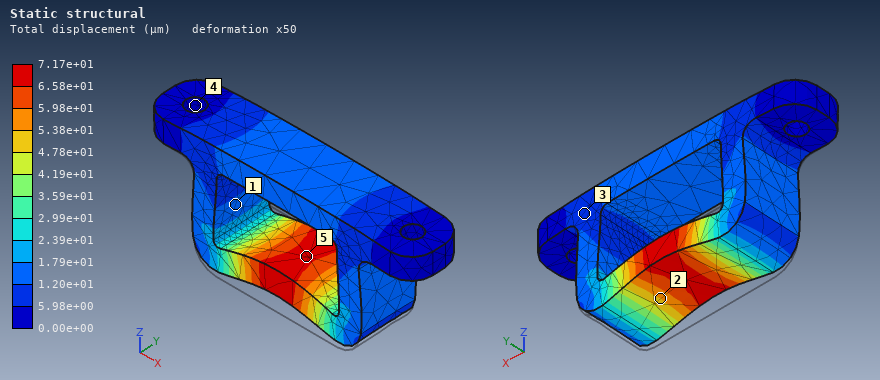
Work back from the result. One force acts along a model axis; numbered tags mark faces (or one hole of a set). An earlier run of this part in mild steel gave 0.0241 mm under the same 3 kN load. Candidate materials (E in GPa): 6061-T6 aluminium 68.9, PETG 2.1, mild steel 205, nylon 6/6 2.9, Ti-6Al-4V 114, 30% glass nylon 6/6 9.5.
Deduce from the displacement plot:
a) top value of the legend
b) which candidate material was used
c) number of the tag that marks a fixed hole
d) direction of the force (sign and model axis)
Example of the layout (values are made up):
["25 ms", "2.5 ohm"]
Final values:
["7.17e+01 µm", "6061-T6 aluminium", "4", "+Z"]
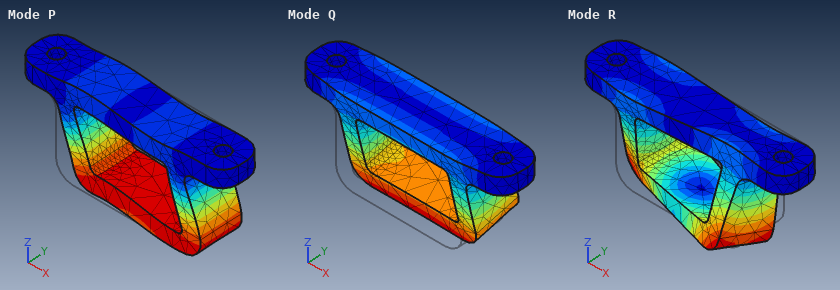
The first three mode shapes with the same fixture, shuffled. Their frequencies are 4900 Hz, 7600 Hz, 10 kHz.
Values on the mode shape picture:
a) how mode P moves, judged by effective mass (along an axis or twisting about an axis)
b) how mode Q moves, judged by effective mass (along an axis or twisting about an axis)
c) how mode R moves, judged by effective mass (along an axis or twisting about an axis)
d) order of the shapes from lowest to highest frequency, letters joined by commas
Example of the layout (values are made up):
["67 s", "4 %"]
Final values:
["along X", "along Y", "twisting about Z", "Q, P, R"]
